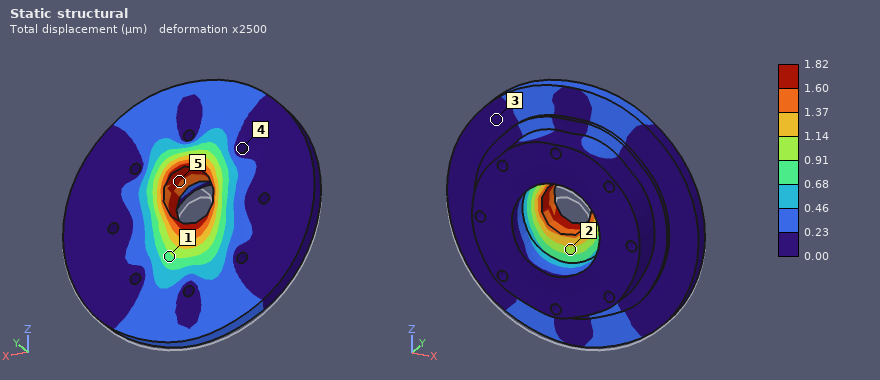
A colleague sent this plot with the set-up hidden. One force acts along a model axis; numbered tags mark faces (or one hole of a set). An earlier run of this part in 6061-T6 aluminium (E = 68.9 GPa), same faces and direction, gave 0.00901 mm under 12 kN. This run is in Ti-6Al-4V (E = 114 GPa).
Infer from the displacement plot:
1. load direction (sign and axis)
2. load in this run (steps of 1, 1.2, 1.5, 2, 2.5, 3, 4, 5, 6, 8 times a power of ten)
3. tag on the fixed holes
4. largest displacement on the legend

+Z
4 kN
4
1.82 µm
